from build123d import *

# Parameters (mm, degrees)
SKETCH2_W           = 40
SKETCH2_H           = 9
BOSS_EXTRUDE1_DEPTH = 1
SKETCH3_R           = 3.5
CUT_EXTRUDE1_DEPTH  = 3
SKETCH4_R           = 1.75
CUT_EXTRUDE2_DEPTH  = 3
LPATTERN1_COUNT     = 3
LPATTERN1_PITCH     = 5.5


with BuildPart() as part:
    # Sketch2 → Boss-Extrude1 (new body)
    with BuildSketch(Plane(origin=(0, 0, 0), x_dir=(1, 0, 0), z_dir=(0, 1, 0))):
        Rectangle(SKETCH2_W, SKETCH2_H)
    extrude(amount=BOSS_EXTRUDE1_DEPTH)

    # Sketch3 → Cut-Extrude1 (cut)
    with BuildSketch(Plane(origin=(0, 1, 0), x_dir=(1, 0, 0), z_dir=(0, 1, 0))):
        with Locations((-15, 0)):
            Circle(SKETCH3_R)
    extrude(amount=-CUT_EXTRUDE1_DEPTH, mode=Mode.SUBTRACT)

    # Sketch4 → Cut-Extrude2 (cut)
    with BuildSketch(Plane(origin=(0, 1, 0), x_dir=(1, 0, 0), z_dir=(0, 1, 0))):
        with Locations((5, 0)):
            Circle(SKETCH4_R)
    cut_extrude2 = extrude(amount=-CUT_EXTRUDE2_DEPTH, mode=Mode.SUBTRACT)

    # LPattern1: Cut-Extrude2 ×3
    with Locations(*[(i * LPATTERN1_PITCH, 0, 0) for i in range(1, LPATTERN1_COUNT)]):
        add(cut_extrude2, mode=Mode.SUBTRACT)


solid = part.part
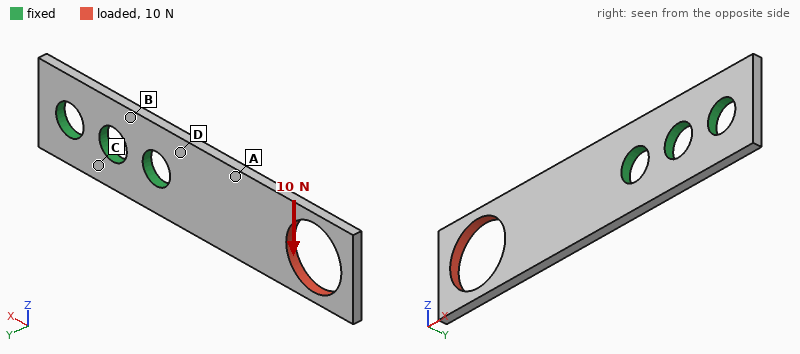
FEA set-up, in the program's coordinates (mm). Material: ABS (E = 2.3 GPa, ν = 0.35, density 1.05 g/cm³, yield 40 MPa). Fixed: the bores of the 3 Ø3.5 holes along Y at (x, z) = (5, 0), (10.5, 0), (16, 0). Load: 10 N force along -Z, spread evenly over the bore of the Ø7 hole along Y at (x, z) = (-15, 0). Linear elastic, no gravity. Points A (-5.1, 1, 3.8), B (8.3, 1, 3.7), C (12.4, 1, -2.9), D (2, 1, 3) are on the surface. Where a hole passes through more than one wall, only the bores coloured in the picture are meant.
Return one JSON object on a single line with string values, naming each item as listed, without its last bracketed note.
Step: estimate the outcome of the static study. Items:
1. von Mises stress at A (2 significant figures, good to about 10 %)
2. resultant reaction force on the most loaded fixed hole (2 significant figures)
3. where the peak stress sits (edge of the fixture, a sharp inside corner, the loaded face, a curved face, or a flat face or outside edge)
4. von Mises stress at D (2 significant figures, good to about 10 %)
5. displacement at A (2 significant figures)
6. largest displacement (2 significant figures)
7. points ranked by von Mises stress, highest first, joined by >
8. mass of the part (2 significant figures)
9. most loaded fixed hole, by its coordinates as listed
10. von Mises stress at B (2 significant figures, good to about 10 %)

{"von Mises stress at A": "6.2 MPa", "resultant reaction force on the most loaded fixed hole": "20 N", "where the peak stress sits": "edge of the fixture", "von Mises stress at D": "8.4 MPa", "displacement at A": "0.11 mm", "largest displacement": "0.47 mm", "points ranked by von Mises stress, highest first, joined by >": "D > A > B > C", "mass of the part": "0.31 g", "most loaded fixed hole, by its coordinates as listed": "(5, 0)", "von Mises stress at B": "3.4 MPa"}
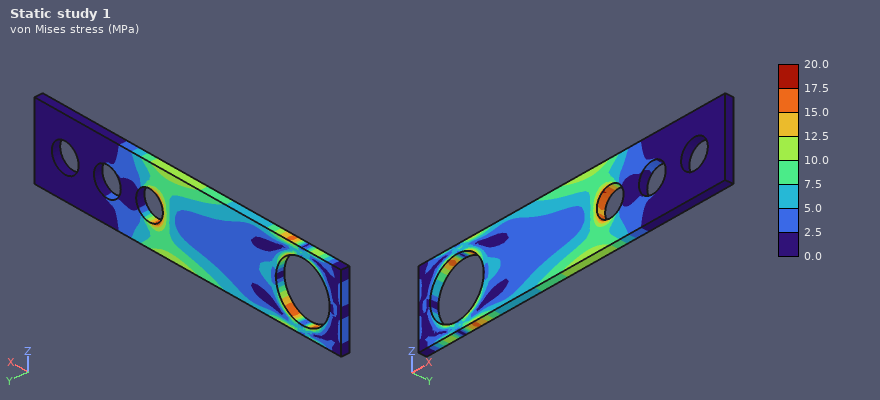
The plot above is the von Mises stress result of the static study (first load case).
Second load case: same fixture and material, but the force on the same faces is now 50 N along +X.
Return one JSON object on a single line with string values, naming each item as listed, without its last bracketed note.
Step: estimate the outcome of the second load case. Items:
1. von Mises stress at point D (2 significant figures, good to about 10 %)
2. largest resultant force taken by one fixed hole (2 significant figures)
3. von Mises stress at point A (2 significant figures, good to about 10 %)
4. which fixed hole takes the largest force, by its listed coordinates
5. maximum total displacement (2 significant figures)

{"von Mises stress at point D": "4.6 MPa", "largest resultant force taken by one fixed hole": "44 N", "von Mises stress at point A": "6.1 MPa", "which fixed hole takes the largest force, by its listed coordinates": "(5, 0)", "maximum total displacement": "0.15 mm"}
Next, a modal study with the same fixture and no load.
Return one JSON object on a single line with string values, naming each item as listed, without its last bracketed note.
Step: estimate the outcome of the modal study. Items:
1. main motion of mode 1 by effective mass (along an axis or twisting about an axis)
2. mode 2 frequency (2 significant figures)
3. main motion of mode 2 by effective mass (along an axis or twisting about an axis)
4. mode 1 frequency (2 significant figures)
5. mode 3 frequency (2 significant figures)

{"main motion of mode 1 by effective mass": "along Y", "mode 2 frequency": "2100 Hz", "main motion of mode 2 by effective mass": "twisting about X", "mode 1 frequency": "540 Hz", "mode 3 frequency": "2300 Hz"}
